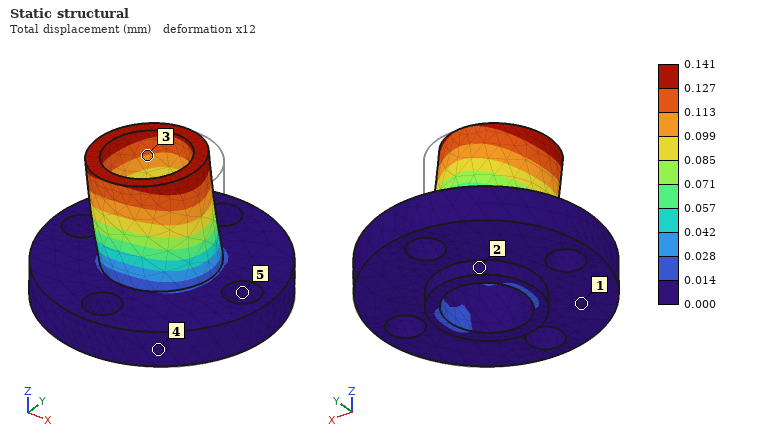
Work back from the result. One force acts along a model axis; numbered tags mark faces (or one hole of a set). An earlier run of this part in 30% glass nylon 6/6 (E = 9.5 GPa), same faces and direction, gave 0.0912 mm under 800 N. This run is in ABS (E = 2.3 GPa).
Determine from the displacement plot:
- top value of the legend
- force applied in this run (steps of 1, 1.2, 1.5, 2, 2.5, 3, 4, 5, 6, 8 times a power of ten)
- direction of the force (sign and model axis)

0.141 mm
300 N
-X
